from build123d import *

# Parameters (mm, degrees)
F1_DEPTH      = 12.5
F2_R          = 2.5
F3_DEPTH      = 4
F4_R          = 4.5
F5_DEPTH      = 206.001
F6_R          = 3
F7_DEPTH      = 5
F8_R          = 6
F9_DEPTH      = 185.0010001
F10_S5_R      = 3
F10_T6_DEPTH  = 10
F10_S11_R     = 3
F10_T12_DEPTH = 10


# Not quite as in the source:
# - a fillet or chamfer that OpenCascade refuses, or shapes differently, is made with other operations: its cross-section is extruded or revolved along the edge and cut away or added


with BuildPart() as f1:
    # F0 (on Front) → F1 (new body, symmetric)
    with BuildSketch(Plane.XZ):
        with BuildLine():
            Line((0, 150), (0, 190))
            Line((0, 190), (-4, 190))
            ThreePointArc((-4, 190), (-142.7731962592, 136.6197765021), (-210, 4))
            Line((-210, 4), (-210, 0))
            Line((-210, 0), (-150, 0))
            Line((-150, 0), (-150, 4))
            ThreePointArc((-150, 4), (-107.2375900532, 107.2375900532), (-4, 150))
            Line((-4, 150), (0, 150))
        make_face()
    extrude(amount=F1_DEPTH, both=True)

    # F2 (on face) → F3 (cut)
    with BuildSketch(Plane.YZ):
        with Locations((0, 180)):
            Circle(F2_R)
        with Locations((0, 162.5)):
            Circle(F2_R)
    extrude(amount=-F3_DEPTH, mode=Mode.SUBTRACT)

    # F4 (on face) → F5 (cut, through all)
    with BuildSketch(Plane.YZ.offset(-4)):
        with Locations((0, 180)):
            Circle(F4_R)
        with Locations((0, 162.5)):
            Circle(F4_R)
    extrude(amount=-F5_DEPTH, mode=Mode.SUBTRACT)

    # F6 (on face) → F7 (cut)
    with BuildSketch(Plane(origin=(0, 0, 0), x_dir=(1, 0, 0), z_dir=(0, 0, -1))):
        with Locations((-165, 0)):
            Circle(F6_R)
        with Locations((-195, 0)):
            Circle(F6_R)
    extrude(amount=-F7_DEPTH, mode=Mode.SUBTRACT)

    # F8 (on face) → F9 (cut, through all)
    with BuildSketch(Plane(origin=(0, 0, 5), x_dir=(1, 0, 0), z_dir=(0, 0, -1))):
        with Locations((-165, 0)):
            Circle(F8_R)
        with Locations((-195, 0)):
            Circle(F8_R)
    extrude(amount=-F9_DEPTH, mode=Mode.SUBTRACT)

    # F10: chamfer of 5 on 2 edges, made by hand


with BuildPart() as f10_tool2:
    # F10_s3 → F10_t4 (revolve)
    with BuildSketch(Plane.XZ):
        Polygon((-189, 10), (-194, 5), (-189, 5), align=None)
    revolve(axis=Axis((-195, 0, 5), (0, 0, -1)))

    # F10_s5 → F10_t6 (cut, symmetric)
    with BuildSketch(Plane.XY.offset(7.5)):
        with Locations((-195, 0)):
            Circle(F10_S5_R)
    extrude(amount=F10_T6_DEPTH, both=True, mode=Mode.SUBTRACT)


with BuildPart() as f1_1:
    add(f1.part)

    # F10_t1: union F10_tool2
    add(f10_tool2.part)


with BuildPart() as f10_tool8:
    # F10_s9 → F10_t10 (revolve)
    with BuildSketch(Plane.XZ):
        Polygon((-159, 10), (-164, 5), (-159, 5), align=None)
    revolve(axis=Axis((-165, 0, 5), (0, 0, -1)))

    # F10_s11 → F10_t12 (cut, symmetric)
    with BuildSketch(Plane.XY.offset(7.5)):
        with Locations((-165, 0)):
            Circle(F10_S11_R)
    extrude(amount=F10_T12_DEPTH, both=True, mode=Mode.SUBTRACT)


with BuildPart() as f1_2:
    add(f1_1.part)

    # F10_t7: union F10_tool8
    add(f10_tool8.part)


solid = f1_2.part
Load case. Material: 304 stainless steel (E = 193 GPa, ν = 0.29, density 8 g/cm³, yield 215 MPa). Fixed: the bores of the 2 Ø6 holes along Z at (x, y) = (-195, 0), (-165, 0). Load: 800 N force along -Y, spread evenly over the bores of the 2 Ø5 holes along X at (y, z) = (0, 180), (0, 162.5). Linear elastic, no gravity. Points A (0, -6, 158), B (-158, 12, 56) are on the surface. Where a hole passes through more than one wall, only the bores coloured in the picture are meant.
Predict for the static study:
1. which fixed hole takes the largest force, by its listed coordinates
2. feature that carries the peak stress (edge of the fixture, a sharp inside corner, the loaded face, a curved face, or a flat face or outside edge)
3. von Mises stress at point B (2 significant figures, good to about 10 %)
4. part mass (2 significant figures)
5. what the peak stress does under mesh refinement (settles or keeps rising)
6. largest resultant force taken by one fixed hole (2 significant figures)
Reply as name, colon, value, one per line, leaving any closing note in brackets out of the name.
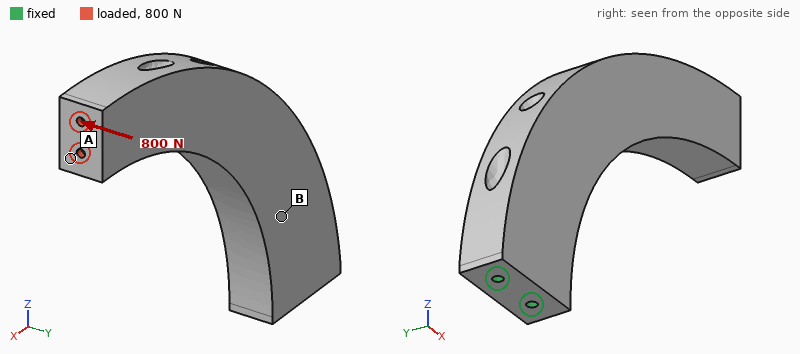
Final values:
which fixed hole takes the largest force, by its listed coordinates: (-165, 0)
feature that carries the peak stress: edge of the fixture
von Mises stress at point B: 33 MPa
part mass: 2.4 kg
what the peak stress does under mesh refinement: keeps rising
largest resultant force taken by one fixed hole: 4.4 kN
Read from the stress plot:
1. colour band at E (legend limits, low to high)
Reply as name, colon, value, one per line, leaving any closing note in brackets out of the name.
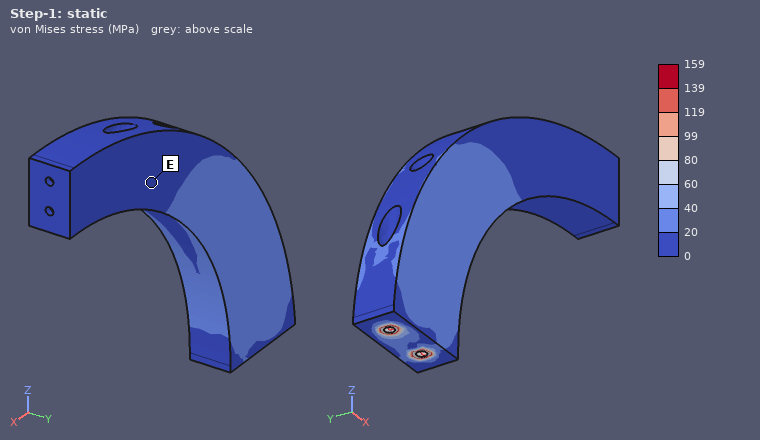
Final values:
colour band at E: 0 to 20 MPa
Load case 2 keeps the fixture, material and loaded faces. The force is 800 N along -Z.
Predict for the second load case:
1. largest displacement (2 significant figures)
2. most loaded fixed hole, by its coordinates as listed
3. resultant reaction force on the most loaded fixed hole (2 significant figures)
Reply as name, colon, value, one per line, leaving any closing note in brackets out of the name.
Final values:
largest displacement: 0.12 mm
most loaded fixed hole, by its coordinates as listed: (-165, 0)
resultant reaction force on the most loaded fixed hole: 4.6 kN
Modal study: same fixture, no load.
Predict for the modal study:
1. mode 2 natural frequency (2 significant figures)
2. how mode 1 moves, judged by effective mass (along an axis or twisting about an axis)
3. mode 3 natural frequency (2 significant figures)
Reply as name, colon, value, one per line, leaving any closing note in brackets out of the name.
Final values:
mode 2 natural frequency: 520 Hz
how mode 1 moves, judged by effective mass: along Y
mode 3 natural frequency: 1000 Hz
